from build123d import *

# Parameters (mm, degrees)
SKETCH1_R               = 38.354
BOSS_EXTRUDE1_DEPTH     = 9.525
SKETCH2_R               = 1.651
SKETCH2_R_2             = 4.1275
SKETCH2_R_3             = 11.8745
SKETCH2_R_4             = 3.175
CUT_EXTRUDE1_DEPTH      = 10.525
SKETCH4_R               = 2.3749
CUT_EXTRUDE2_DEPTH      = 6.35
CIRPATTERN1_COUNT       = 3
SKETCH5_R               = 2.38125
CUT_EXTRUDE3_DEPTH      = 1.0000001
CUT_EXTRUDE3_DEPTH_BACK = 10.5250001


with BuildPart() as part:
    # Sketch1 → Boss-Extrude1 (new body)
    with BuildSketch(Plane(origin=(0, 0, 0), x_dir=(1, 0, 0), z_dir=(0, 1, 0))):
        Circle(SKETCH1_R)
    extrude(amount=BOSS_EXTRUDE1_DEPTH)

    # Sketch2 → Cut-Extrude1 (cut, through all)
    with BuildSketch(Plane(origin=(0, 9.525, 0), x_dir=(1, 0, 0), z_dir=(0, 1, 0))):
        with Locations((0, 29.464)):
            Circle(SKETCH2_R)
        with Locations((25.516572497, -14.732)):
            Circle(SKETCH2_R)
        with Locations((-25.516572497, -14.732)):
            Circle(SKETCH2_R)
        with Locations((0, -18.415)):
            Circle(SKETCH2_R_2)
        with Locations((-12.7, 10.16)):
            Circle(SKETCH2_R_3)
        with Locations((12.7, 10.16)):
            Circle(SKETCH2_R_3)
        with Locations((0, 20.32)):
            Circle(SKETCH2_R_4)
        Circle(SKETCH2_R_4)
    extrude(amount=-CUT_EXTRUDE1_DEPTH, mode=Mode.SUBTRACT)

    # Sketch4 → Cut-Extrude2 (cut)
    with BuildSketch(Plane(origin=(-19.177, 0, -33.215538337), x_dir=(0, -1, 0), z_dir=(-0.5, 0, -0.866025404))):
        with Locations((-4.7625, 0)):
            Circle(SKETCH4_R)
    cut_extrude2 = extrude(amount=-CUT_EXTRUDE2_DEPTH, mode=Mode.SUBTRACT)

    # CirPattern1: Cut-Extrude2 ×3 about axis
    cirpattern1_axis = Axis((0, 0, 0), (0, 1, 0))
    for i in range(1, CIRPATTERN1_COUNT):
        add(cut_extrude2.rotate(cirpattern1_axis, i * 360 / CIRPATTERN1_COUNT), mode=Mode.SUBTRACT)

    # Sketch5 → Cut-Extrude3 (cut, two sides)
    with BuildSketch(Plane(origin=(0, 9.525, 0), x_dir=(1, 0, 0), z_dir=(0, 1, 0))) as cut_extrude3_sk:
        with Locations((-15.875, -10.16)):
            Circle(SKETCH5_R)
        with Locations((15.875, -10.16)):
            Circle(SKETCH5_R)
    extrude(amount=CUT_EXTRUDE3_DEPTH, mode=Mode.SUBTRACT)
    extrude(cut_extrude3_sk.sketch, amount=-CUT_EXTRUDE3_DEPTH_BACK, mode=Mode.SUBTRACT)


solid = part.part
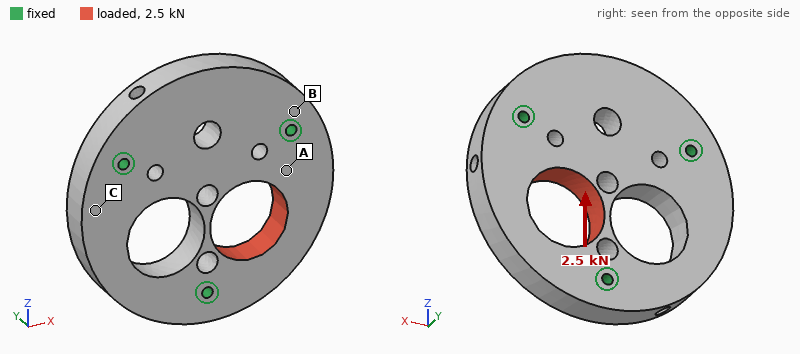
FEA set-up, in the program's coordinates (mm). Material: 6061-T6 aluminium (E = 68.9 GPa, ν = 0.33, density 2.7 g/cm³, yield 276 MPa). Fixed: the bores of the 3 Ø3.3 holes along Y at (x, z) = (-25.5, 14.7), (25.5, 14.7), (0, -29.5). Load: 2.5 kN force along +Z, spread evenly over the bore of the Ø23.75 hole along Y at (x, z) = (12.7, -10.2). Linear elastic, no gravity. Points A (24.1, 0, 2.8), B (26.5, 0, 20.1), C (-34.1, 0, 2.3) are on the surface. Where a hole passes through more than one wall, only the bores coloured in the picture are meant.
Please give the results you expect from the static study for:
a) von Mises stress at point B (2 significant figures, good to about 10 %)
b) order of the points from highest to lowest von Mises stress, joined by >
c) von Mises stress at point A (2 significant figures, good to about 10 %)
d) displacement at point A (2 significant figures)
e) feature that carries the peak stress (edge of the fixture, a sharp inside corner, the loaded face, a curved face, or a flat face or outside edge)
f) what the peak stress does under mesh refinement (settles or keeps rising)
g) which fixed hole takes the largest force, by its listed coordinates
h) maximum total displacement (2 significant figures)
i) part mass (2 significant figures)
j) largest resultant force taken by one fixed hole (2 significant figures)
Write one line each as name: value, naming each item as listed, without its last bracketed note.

von Mises stress at point B: 5.1 MPa
order of the points from highest to lowest von Mises stress, joined by >: A > B > C
von Mises stress at point A: 8.8 MPa
displacement at point A: 1.7 µm
feature that carries the peak stress: edge of the fixture
what the peak stress does under mesh refinement: keeps rising
which fixed hole takes the largest force, by its listed coordinates: (25.5, 14.7)
maximum total displacement: 5.0 µm
part mass: 91 g
largest resultant force taken by one fixed hole: 1.5 kN
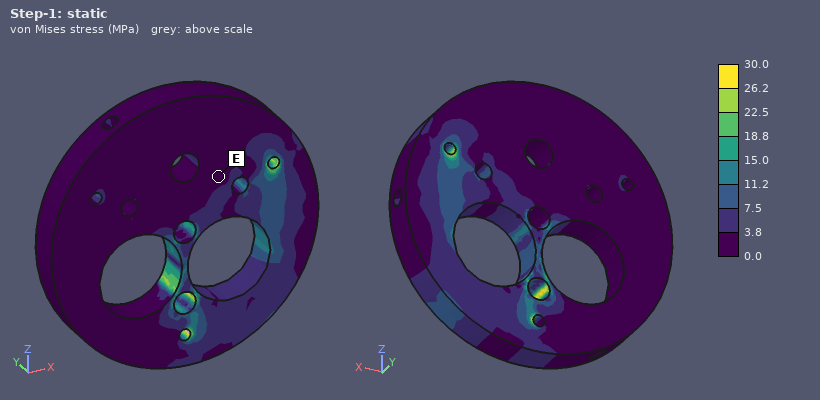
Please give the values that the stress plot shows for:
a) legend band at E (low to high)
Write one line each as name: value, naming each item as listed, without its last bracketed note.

legend band at E: 0.0 to 3.8 MPa
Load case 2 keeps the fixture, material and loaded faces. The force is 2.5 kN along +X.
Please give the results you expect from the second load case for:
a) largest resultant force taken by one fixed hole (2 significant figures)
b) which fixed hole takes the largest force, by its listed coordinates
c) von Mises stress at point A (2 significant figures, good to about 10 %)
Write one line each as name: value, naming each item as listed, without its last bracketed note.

largest resultant force taken by one fixed hole: 1.3 kN
which fixed hole takes the largest force, by its listed coordinates: (0, -29.5)
von Mises stress at point A: 4.0 MPa
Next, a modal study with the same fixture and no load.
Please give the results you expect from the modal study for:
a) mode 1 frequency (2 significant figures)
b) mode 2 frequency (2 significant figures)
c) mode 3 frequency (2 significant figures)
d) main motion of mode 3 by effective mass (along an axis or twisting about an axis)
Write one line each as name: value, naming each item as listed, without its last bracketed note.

mode 1 frequency: 8400 Hz
mode 2 frequency: 8700 Hz
mode 3 frequency: 10 kHz
main motion of mode 3 by effective mass: along Y
